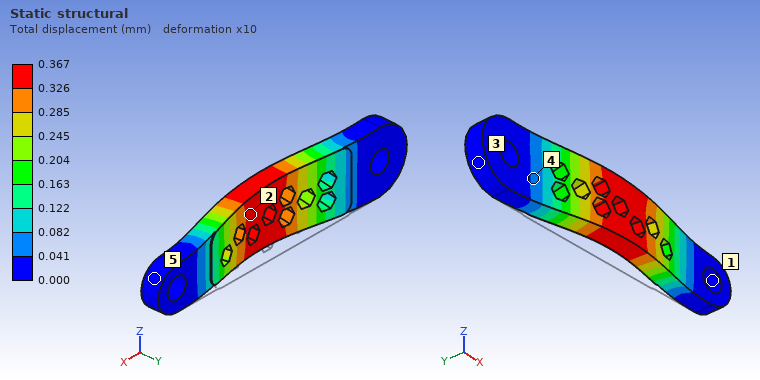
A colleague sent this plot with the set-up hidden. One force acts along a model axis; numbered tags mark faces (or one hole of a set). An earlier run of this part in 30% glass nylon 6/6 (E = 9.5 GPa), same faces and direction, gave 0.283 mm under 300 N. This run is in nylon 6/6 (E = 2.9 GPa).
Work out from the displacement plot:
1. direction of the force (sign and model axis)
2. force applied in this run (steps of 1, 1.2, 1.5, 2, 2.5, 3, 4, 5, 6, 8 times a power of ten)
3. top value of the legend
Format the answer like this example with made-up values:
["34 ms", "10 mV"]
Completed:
["-Y", "120 N", "0.367 mm"]
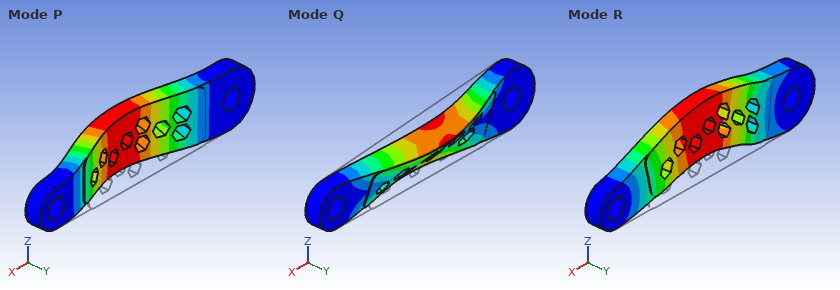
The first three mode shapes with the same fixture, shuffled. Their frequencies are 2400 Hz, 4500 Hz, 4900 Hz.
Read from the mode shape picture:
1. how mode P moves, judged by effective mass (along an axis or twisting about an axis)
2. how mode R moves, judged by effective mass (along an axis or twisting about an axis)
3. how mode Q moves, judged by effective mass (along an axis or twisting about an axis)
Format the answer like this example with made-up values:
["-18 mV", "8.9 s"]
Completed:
["along Y", "along Z", "twisting about X"]
